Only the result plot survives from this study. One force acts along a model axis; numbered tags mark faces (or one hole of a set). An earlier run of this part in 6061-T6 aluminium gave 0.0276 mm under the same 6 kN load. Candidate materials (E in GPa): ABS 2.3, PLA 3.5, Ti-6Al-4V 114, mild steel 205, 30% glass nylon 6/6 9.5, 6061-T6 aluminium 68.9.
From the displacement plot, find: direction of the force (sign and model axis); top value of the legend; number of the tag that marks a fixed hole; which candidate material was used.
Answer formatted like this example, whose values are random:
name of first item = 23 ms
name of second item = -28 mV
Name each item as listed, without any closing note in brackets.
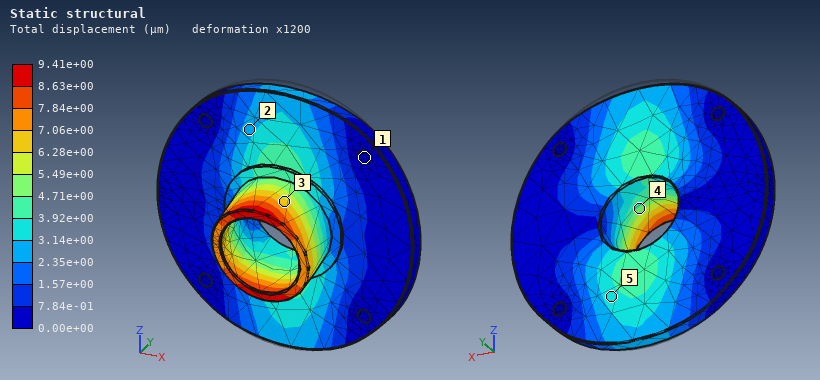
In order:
direction of the force = -Z
top value of the legend = 9.41e+00 µm
number of the tag that marks a fixed hole = 1
which candidate material was used = mild steel
